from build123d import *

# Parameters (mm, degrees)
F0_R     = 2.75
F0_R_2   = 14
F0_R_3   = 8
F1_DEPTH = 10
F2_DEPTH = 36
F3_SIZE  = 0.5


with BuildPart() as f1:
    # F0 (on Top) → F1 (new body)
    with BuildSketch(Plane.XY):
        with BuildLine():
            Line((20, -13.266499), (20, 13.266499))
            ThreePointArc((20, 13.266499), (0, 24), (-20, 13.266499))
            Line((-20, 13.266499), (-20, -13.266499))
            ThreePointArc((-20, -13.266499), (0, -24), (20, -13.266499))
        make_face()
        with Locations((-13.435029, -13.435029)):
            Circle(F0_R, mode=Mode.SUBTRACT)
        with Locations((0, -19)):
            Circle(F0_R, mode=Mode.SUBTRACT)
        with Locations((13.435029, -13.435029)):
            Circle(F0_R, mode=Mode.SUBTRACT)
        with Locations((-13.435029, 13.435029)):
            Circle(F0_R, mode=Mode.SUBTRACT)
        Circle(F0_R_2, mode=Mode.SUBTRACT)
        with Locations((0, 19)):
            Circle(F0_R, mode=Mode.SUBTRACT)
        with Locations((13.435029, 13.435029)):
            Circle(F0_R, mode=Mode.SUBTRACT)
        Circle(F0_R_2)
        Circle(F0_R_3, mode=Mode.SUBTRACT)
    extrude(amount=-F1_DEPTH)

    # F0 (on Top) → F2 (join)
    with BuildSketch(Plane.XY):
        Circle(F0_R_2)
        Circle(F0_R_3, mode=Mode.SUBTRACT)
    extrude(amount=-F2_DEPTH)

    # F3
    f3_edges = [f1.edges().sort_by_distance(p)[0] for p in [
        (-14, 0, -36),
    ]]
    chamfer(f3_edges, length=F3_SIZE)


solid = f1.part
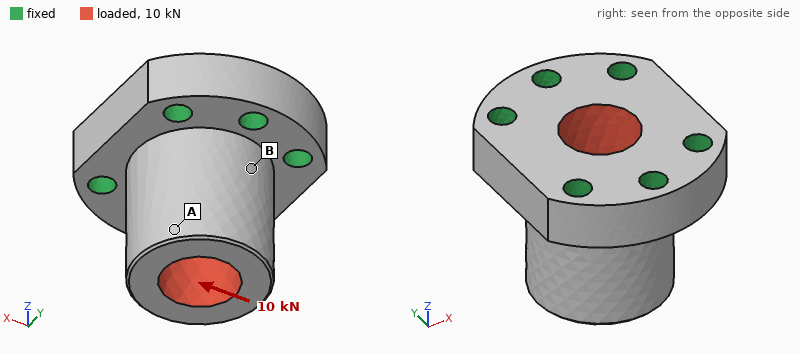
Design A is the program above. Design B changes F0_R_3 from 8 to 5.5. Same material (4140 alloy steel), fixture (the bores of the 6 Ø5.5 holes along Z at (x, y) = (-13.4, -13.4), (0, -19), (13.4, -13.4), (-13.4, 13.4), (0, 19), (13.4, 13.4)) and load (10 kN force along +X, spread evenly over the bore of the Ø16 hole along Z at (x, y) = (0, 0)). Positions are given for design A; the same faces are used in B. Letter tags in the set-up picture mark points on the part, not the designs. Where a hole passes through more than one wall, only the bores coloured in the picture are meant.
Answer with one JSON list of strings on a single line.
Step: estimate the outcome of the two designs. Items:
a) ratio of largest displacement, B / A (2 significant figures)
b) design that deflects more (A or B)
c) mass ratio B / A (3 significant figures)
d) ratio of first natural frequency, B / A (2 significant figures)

["0.86", "A", "1.16", "0.97"]
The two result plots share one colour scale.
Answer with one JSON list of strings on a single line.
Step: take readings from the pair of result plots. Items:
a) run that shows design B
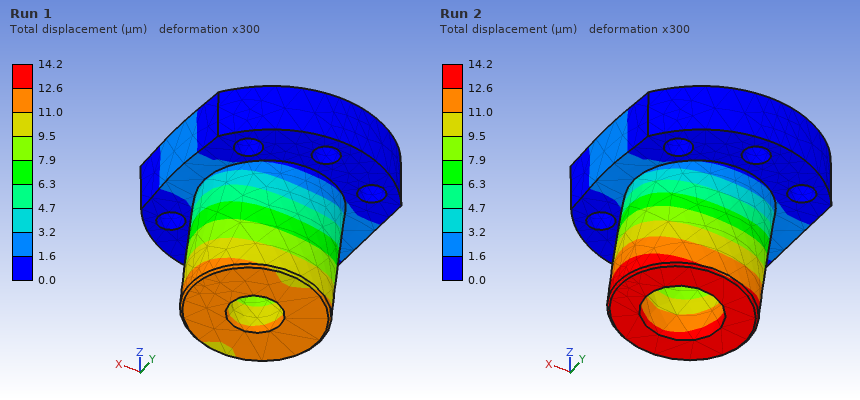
["Run 1"]
